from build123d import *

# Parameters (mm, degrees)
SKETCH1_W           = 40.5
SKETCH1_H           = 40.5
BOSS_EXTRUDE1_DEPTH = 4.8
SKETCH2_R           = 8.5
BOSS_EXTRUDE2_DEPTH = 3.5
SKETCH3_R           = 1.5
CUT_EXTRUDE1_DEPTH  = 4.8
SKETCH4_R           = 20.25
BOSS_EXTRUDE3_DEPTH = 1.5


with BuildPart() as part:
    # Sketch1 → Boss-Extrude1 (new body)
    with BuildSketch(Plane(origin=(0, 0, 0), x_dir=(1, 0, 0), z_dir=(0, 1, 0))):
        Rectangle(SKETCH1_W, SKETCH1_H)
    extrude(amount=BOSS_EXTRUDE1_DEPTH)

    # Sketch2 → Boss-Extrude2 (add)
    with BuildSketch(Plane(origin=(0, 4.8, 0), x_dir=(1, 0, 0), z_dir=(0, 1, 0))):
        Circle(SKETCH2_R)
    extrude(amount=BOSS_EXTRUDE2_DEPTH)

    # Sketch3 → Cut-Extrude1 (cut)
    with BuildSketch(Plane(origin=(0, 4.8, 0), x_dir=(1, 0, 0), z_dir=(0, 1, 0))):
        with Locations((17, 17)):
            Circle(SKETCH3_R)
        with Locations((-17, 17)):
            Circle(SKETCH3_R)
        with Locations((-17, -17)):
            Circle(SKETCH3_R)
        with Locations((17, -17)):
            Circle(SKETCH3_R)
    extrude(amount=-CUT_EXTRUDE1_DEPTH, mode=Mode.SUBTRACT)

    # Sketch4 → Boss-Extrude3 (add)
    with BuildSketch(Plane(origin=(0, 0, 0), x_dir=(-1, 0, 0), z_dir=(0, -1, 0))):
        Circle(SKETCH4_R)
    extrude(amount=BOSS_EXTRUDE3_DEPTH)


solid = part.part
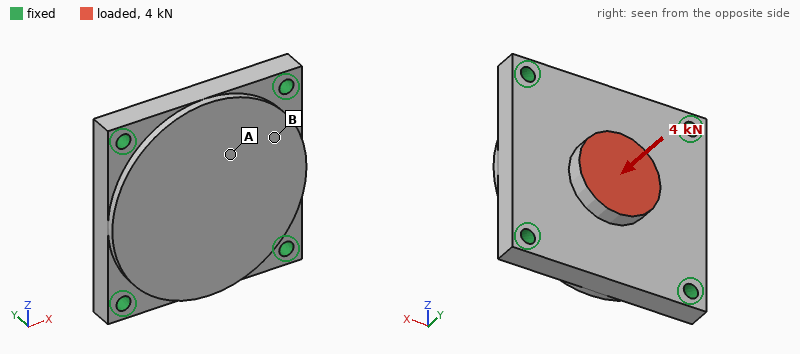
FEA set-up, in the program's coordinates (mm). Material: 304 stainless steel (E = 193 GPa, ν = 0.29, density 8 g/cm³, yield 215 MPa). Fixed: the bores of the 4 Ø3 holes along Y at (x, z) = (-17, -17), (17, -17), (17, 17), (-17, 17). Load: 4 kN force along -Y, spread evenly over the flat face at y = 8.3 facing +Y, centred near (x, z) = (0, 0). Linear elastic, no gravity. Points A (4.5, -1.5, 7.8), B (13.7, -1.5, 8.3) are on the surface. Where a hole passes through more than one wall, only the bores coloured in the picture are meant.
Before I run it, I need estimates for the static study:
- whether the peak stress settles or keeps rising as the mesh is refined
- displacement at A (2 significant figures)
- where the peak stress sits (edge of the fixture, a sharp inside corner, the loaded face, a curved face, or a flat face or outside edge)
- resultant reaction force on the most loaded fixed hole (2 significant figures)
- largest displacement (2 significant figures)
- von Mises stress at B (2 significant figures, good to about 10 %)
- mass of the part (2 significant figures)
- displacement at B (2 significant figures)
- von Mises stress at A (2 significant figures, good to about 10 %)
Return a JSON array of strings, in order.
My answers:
["keeps rising", "12 µm", "edge of the fixture", "1.1 kN", "14 µm", "27 MPa", "84 g", "7.5 µm", "54 MPa"]
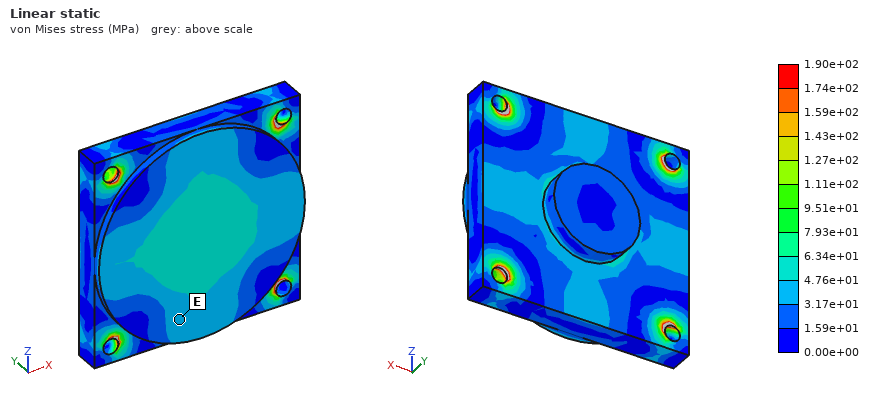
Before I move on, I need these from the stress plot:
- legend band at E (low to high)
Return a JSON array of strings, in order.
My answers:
["3.17e+01 to 4.76e+01 MPa"]
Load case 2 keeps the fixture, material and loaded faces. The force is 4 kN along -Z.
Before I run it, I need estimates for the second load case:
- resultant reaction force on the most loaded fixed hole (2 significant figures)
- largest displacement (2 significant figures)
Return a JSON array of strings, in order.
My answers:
["1.1 kN", "7.9 µm"]
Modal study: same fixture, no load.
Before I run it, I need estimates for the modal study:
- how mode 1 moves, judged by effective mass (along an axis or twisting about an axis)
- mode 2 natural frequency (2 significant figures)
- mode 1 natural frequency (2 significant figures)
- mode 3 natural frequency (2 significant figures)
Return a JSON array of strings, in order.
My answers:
["along Y", "22 kHz", "13 kHz", "22 kHz"]
